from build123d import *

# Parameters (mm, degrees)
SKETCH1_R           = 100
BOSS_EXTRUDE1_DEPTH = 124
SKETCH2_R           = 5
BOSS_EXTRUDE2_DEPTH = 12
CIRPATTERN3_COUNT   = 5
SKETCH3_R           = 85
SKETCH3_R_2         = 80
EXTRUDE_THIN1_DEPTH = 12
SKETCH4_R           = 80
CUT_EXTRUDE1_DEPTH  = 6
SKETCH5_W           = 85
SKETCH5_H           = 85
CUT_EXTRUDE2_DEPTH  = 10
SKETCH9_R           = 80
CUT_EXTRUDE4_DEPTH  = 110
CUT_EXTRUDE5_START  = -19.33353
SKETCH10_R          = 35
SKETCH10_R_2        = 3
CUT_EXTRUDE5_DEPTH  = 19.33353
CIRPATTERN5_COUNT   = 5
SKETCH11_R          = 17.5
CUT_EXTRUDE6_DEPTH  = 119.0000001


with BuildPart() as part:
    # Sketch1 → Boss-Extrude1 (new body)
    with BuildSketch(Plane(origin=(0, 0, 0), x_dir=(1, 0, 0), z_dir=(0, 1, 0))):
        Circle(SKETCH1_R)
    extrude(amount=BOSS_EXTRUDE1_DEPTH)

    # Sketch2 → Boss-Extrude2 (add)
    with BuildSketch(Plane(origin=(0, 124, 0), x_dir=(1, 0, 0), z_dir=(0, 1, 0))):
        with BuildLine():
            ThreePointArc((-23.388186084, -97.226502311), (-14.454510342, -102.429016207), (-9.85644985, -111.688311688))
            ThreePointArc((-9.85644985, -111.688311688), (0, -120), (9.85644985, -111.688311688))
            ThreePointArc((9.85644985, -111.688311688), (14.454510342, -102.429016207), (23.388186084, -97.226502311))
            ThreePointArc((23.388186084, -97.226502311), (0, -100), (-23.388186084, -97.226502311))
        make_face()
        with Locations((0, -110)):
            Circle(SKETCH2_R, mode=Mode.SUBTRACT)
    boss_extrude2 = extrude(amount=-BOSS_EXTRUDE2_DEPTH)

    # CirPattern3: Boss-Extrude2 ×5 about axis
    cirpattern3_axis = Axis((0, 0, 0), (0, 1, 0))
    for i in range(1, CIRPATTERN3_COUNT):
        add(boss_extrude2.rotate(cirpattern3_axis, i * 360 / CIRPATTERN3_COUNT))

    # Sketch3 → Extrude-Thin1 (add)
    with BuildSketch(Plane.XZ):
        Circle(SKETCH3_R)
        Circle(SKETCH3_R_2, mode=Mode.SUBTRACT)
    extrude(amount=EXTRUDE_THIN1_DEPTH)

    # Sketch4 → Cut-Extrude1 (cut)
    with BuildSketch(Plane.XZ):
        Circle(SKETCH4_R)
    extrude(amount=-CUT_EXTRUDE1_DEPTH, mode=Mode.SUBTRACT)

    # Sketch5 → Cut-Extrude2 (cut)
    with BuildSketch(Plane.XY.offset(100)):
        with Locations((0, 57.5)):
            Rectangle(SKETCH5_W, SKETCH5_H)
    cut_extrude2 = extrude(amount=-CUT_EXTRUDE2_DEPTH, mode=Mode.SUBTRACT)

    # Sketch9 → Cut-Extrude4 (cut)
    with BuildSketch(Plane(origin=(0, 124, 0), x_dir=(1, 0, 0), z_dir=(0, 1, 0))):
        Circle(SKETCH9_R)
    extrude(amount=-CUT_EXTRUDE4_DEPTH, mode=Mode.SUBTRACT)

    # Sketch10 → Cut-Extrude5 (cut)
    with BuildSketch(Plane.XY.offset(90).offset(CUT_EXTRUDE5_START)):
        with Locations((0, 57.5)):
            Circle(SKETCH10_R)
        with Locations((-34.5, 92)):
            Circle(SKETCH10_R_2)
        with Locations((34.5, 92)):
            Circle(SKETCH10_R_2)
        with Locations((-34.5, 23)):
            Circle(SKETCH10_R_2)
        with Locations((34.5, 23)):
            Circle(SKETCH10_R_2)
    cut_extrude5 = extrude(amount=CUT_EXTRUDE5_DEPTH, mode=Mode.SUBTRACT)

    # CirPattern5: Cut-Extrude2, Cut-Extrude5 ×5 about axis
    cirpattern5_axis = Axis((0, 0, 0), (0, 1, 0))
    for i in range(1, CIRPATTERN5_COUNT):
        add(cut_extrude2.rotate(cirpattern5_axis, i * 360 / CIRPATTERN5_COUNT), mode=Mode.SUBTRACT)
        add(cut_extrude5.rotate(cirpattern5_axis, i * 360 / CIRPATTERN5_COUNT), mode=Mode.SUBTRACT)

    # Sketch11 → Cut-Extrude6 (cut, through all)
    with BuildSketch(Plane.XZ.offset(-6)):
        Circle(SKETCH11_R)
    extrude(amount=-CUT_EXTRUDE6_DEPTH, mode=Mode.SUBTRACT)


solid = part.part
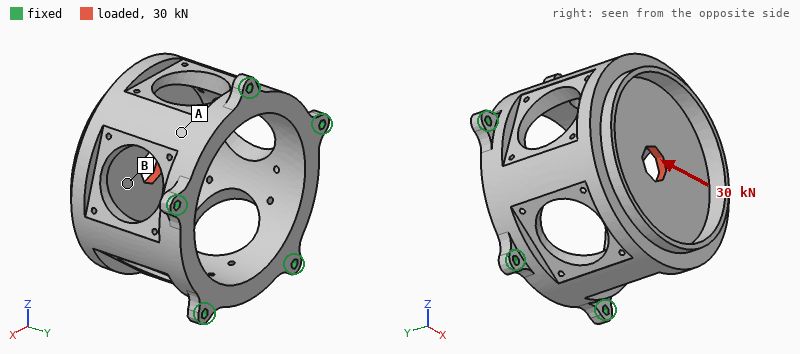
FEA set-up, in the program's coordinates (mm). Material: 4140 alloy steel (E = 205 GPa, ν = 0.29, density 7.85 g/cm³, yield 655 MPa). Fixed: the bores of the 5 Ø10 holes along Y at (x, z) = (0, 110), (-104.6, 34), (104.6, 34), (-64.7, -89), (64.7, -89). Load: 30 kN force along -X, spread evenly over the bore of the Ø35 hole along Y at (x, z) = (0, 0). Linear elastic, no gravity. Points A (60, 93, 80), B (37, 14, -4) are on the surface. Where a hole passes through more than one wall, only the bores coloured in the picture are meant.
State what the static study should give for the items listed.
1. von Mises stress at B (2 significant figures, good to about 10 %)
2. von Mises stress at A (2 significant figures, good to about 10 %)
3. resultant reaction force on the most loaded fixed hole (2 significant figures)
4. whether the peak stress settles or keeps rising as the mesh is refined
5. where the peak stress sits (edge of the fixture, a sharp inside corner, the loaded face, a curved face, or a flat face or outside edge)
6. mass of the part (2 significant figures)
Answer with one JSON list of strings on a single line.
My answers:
["29 MPa", "12 MPa", "14 kN", "keeps rising", "edge of the fixture", "8.8 kg"]
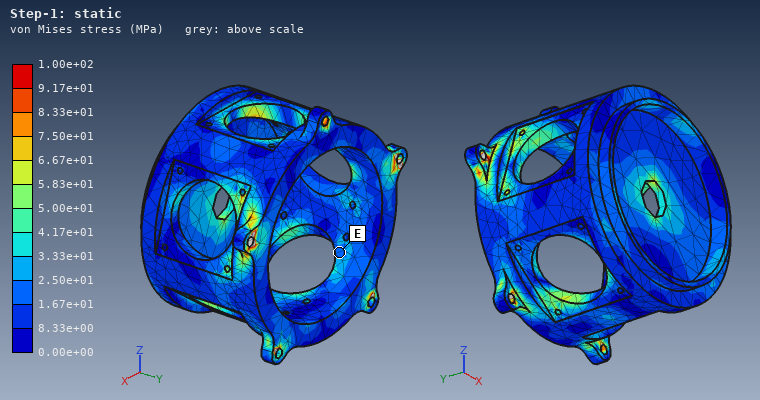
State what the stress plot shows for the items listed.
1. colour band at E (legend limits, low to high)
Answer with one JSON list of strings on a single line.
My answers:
["1.67e+01 to 2.50e+01 MPa"]
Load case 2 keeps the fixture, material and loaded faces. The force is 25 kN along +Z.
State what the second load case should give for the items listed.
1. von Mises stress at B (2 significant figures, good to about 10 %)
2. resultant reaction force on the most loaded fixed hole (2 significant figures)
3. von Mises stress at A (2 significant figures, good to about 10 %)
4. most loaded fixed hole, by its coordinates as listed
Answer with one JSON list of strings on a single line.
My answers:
["16 MPa", "12 kN", "12 MPa", "(0, 110)"]
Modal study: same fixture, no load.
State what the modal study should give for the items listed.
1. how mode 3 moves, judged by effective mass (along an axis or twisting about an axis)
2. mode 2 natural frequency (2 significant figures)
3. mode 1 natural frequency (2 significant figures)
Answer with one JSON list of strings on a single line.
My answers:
["along Y", "1600 Hz", "1600 Hz"]
